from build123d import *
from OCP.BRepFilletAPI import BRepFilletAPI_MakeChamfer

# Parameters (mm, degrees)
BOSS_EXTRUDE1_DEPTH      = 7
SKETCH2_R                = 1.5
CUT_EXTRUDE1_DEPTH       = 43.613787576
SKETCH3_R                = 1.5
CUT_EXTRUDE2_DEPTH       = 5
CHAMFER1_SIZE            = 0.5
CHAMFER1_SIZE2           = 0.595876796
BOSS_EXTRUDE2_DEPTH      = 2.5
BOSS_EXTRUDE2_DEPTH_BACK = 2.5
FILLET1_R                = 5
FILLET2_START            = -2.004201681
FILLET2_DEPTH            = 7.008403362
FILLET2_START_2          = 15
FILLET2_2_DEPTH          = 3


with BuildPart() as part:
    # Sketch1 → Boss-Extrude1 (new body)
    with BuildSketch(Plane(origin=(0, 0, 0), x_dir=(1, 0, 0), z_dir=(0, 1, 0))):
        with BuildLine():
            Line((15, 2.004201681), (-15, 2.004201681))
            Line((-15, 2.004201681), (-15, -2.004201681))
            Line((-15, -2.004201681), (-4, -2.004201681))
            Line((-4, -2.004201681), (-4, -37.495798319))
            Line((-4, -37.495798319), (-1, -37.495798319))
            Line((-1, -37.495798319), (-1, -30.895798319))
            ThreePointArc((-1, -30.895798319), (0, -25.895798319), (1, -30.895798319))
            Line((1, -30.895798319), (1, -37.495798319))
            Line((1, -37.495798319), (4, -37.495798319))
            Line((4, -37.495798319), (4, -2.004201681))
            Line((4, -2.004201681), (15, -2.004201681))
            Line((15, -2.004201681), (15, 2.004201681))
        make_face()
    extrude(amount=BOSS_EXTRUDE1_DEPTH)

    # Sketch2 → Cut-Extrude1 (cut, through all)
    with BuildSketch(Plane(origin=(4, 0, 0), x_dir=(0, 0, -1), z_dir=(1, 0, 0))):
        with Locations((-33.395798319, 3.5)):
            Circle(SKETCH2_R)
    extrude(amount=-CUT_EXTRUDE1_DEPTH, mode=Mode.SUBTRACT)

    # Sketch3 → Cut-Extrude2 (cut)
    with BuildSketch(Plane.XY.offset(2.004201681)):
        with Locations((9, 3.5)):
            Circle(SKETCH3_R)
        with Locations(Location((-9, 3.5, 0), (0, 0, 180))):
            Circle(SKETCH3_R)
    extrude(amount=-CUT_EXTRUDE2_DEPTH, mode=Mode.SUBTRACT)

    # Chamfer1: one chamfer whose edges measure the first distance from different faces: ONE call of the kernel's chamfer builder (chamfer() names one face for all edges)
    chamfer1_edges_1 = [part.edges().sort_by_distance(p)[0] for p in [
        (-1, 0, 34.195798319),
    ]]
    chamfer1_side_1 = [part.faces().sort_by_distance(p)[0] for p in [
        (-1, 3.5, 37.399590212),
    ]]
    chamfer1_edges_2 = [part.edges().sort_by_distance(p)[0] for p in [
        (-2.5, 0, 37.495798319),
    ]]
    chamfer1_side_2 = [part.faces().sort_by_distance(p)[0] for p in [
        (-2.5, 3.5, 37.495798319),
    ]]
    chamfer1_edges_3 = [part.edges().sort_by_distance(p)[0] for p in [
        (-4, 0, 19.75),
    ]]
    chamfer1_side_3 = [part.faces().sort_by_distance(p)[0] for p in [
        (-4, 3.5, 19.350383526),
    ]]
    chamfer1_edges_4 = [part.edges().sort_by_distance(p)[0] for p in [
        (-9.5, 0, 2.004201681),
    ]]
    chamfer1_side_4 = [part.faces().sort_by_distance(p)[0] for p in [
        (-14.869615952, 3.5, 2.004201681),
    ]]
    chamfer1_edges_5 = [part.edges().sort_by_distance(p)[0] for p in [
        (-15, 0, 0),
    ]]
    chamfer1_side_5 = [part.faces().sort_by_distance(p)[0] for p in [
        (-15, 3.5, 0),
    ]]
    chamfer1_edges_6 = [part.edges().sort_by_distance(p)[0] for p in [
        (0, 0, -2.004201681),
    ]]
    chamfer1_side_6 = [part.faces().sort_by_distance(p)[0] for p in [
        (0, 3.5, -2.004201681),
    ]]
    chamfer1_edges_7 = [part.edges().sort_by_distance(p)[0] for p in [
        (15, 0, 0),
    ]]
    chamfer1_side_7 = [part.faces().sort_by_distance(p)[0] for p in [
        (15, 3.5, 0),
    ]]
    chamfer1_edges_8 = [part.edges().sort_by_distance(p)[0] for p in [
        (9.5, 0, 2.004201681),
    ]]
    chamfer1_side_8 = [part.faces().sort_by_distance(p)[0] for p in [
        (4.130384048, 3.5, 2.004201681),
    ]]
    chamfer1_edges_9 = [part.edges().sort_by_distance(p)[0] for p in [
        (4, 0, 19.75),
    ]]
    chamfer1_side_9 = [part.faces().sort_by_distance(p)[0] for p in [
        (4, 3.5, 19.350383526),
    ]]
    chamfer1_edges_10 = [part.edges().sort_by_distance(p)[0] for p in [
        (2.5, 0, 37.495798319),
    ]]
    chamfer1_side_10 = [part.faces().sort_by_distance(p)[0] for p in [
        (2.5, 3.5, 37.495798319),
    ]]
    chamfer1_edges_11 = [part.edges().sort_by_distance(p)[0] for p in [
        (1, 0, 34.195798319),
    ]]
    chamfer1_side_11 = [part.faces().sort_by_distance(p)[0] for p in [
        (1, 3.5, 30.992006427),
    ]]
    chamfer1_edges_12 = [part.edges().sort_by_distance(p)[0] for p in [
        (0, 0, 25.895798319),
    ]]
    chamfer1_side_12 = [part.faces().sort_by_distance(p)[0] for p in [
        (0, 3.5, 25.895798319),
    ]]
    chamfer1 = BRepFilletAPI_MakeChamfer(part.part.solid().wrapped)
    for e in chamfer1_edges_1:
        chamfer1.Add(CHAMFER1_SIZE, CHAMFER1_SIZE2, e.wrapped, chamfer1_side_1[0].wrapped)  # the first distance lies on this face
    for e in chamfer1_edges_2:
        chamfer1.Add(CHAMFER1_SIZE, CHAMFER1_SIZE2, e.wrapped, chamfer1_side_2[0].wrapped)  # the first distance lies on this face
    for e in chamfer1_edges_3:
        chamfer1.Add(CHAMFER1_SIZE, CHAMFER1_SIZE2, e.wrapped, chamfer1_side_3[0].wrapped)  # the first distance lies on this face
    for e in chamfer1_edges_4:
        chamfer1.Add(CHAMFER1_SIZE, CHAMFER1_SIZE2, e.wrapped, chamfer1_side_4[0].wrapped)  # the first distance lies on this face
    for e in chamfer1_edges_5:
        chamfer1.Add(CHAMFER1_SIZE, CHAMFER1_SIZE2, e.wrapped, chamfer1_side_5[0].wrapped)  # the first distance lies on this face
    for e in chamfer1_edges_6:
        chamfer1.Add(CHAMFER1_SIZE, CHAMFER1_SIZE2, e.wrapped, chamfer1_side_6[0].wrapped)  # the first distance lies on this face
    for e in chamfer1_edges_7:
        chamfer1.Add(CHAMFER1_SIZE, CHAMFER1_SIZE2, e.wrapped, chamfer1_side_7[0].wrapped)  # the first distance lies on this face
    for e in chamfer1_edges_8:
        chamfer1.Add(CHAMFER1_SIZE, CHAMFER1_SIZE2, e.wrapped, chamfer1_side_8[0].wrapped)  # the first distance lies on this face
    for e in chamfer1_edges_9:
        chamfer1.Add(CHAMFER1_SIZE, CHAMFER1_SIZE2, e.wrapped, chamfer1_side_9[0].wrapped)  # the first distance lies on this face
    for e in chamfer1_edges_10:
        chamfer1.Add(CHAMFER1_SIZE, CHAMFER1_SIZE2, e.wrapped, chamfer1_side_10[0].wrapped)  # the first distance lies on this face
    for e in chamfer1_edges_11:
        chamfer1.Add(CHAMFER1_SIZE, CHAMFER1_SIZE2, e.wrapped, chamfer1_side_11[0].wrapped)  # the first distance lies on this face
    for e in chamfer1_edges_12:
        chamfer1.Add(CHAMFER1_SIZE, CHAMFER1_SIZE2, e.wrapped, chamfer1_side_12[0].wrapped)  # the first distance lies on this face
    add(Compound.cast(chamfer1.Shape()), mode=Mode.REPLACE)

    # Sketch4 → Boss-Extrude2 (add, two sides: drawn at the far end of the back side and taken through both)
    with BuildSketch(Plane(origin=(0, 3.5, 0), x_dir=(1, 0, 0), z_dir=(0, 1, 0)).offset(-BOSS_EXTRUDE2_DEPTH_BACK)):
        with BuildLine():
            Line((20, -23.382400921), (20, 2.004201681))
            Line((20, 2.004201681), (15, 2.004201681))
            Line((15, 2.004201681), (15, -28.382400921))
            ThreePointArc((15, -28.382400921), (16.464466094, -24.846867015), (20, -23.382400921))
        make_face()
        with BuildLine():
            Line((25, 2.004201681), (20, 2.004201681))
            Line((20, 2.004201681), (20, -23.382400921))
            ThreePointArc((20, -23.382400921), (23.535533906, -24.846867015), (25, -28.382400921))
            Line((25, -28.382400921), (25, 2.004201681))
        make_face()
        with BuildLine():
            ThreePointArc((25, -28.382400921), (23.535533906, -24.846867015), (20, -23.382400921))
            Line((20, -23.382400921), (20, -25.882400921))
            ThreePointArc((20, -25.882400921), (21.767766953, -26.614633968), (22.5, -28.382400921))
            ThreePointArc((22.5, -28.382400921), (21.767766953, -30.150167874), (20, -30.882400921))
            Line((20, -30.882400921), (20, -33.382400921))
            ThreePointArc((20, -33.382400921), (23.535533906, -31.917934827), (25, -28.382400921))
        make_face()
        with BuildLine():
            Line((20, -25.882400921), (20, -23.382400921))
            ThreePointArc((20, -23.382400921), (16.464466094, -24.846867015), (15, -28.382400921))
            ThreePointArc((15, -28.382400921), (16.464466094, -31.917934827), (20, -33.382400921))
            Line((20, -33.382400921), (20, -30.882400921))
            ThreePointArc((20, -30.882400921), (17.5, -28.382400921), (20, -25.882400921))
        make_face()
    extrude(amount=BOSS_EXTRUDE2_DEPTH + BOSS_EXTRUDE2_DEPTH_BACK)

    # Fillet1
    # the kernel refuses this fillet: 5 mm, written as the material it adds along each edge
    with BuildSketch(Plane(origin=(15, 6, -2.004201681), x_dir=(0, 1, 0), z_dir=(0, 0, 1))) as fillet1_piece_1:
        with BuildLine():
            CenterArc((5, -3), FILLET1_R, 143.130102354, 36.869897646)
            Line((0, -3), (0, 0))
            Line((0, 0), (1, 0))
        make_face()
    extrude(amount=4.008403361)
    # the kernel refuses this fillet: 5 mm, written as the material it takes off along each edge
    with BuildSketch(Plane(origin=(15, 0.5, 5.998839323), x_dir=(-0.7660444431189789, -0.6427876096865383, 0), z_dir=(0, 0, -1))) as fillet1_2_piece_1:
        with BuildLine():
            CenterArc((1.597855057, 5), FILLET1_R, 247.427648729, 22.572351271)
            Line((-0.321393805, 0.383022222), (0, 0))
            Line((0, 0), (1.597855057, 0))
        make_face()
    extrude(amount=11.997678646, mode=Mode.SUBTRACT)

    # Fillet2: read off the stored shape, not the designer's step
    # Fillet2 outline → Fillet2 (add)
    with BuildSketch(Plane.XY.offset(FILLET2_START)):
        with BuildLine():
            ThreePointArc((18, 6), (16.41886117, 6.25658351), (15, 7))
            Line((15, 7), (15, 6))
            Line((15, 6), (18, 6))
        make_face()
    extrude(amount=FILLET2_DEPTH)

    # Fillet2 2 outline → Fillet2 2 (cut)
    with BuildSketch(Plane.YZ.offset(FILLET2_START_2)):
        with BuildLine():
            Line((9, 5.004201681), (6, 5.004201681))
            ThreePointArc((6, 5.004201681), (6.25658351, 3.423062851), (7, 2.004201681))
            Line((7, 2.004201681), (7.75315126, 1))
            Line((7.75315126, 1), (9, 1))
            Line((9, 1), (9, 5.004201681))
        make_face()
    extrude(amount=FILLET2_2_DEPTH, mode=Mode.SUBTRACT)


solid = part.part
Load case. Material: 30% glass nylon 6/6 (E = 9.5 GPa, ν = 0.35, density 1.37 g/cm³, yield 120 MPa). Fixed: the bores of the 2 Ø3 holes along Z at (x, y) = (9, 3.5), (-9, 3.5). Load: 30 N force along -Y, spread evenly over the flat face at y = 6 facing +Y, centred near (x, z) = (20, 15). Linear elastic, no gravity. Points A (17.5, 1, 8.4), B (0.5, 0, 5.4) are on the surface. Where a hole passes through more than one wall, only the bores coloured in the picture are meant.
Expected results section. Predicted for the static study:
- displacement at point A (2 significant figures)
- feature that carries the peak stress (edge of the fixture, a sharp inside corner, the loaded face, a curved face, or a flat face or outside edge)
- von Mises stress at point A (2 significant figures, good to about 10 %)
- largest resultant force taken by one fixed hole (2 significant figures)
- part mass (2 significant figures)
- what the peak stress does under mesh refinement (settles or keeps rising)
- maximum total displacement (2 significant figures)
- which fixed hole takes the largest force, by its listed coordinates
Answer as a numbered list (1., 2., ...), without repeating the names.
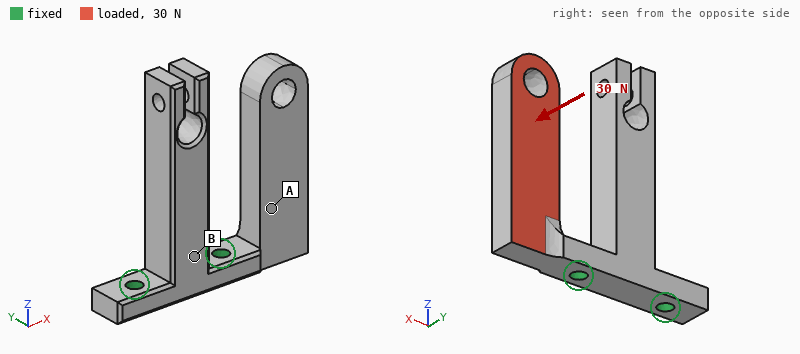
1. 0.10 mm
2. a sharp inside corner
3. 6.4 MPa
4. 35 N
5. 5.6 g
6. keeps rising
7. 0.43 mm
8. (9, 3.5)
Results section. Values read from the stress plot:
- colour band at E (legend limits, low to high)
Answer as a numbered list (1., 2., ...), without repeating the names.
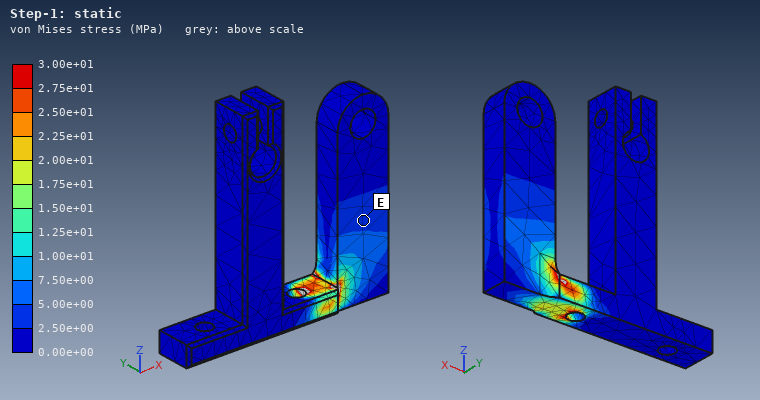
1. 2.50e+00 to 5.00e+00 MPa
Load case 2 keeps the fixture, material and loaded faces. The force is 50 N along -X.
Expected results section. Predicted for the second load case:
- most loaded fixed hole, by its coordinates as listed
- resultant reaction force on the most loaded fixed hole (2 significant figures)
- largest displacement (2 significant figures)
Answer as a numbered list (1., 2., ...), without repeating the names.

1. (9, 3.5)
2. 48 N
3. 0.66 mm
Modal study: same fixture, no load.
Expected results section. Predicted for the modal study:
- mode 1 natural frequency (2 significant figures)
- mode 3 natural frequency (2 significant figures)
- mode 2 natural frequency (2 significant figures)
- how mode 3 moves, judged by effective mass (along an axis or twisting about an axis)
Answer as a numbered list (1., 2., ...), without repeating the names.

1. 1100 Hz
2. 1600 Hz
3. 1200 Hz
4. along Y
